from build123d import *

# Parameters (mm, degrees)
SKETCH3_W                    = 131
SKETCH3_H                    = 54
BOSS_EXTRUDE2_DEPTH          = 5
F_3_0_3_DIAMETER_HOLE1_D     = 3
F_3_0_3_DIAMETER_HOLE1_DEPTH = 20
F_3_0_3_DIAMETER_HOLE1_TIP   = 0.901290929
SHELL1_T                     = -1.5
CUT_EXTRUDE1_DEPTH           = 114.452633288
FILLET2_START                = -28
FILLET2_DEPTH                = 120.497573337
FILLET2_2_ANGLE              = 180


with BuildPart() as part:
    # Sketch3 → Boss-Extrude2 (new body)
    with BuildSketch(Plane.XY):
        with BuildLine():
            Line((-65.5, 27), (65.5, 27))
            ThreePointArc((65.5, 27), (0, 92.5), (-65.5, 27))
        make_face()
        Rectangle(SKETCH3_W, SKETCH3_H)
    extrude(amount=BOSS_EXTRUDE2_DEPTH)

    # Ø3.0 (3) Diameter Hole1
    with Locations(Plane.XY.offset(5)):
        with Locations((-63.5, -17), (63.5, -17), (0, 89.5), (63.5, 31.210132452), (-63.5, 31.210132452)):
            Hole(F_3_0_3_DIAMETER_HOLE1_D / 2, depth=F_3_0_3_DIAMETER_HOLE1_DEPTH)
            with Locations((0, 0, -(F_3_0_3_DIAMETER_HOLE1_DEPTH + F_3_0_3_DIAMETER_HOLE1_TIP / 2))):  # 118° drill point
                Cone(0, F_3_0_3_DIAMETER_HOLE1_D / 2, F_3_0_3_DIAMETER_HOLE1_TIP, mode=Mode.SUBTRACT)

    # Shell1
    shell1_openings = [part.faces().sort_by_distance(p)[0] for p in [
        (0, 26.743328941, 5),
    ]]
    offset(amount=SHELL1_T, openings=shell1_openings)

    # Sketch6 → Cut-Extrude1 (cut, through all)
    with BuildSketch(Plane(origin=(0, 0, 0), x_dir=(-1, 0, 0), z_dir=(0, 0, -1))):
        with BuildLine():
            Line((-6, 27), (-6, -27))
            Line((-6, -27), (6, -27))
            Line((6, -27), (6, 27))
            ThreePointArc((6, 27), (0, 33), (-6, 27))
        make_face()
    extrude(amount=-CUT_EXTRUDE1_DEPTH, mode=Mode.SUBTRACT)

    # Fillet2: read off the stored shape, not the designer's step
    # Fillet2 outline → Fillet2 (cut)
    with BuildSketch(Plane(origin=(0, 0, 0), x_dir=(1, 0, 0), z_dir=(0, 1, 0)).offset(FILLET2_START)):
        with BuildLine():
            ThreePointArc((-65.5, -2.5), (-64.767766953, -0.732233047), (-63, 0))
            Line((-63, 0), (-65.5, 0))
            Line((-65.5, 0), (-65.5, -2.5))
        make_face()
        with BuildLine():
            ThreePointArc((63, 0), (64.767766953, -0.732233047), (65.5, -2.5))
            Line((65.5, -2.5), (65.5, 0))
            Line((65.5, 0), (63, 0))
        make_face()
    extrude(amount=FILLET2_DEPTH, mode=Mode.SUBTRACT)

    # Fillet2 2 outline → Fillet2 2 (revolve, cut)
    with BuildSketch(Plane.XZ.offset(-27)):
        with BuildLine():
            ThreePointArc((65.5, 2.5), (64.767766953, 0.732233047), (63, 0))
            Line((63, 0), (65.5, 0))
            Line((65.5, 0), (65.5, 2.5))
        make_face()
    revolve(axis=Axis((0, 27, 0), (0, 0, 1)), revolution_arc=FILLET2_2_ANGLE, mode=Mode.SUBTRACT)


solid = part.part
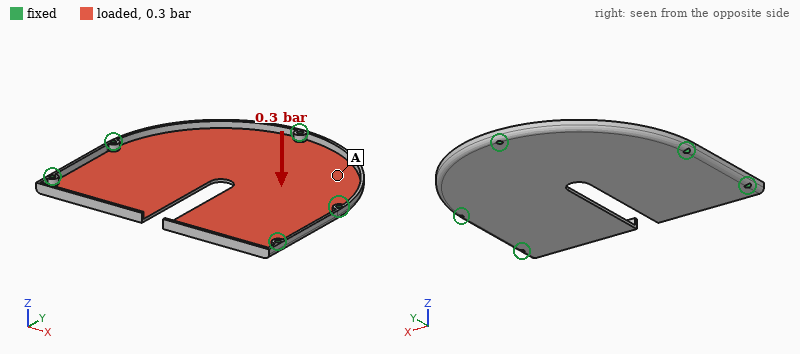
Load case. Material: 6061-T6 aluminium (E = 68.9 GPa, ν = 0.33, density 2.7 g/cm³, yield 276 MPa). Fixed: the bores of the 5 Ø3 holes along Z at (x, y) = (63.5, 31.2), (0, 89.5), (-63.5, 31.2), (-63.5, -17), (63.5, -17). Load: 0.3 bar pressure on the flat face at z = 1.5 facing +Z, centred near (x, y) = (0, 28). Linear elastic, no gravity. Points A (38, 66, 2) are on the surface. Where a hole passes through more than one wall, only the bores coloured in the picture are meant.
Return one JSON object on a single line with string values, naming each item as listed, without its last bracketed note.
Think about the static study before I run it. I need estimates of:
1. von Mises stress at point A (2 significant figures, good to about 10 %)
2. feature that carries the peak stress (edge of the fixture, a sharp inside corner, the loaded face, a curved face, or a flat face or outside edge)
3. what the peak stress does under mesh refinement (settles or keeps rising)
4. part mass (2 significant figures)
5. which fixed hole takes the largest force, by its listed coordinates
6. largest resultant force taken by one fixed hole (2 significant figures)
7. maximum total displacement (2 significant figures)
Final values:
{"von Mises stress at point A": "18 MPa", "feature that carries the peak stress": "edge of the fixture", "what the peak stress does under mesh refinement": "keeps rising", "part mass": "58 g", "which fixed hole takes the largest force, by its listed coordinates": "(0, 89.5)", "largest resultant force taken by one fixed hole": "95 N", "maximum total displacement": "1.1 mm"}
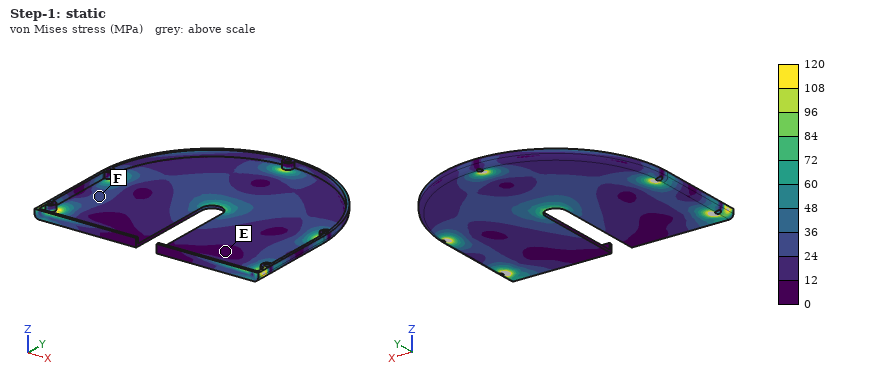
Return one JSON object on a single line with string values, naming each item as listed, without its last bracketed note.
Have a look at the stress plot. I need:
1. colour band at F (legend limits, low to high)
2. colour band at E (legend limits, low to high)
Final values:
{"colour band at F": "24 to 36 MPa", "colour band at E": "0 to 12 MPa"}
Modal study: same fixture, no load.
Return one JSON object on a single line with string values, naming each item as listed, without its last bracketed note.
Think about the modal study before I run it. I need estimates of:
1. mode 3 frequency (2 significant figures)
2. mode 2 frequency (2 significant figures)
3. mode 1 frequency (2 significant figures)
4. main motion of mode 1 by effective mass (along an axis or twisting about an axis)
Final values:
{"mode 3 frequency": "980 Hz", "mode 2 frequency": "700 Hz", "mode 1 frequency": "530 Hz", "main motion of mode 1 by effective mass": "along Z"}
